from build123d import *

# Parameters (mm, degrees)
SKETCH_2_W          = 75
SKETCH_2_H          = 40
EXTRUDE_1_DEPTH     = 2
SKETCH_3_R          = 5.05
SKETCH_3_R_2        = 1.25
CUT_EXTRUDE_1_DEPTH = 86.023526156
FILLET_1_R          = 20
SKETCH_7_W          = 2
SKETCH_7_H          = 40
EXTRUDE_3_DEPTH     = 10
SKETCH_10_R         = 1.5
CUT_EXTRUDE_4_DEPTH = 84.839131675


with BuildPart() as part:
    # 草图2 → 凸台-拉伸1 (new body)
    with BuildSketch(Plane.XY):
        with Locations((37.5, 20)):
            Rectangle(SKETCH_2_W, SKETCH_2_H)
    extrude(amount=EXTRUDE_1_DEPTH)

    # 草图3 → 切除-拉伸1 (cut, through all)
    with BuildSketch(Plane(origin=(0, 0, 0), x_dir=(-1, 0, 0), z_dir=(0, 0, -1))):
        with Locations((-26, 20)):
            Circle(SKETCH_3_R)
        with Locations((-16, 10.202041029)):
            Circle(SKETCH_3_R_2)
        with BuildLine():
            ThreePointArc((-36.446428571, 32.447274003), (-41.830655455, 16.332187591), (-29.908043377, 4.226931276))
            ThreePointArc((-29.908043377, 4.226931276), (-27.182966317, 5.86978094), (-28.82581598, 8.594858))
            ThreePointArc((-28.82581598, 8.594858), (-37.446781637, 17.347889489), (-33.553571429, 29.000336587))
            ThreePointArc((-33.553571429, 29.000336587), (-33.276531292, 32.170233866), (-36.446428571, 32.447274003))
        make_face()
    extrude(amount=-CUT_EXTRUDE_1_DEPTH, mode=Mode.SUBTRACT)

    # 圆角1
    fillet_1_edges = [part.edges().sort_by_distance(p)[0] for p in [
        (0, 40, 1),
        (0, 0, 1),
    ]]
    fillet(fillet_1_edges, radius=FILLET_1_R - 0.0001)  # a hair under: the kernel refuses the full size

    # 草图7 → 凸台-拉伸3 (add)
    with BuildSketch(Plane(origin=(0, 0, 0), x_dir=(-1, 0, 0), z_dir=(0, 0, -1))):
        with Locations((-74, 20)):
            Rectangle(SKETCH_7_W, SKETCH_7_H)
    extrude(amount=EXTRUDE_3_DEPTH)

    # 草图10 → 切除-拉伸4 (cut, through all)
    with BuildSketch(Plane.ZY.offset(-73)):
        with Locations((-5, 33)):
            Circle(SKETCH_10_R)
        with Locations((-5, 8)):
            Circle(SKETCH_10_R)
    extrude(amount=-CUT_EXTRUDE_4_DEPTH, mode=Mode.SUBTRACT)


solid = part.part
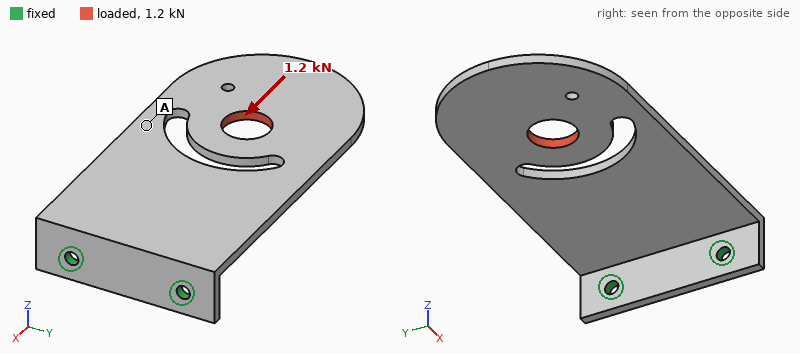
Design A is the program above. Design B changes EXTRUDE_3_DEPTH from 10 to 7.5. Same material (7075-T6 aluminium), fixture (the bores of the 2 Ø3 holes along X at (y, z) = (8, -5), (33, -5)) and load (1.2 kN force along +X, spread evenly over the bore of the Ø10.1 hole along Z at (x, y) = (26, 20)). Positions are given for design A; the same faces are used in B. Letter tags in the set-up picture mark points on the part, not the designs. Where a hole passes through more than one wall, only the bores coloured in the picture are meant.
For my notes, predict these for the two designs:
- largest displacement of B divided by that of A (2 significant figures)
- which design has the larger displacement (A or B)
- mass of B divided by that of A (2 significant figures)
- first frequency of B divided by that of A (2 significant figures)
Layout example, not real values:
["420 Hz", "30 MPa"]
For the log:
["1.1", "B", "0.97", "0.99"]
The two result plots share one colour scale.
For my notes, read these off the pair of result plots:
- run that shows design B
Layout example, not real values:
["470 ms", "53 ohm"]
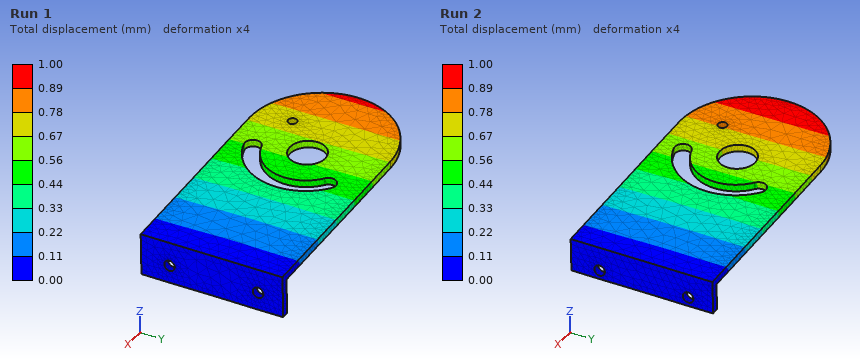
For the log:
["Run 2"]
